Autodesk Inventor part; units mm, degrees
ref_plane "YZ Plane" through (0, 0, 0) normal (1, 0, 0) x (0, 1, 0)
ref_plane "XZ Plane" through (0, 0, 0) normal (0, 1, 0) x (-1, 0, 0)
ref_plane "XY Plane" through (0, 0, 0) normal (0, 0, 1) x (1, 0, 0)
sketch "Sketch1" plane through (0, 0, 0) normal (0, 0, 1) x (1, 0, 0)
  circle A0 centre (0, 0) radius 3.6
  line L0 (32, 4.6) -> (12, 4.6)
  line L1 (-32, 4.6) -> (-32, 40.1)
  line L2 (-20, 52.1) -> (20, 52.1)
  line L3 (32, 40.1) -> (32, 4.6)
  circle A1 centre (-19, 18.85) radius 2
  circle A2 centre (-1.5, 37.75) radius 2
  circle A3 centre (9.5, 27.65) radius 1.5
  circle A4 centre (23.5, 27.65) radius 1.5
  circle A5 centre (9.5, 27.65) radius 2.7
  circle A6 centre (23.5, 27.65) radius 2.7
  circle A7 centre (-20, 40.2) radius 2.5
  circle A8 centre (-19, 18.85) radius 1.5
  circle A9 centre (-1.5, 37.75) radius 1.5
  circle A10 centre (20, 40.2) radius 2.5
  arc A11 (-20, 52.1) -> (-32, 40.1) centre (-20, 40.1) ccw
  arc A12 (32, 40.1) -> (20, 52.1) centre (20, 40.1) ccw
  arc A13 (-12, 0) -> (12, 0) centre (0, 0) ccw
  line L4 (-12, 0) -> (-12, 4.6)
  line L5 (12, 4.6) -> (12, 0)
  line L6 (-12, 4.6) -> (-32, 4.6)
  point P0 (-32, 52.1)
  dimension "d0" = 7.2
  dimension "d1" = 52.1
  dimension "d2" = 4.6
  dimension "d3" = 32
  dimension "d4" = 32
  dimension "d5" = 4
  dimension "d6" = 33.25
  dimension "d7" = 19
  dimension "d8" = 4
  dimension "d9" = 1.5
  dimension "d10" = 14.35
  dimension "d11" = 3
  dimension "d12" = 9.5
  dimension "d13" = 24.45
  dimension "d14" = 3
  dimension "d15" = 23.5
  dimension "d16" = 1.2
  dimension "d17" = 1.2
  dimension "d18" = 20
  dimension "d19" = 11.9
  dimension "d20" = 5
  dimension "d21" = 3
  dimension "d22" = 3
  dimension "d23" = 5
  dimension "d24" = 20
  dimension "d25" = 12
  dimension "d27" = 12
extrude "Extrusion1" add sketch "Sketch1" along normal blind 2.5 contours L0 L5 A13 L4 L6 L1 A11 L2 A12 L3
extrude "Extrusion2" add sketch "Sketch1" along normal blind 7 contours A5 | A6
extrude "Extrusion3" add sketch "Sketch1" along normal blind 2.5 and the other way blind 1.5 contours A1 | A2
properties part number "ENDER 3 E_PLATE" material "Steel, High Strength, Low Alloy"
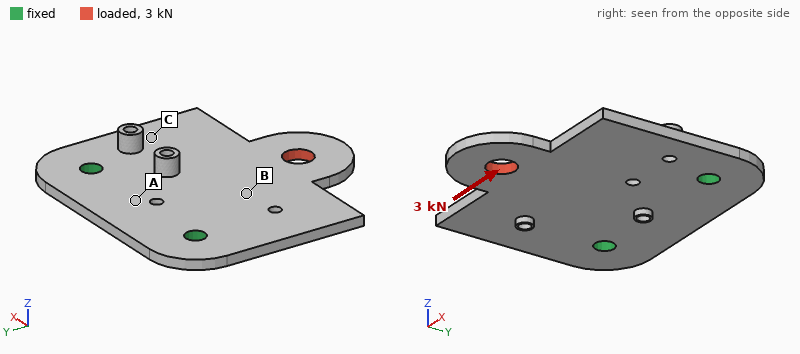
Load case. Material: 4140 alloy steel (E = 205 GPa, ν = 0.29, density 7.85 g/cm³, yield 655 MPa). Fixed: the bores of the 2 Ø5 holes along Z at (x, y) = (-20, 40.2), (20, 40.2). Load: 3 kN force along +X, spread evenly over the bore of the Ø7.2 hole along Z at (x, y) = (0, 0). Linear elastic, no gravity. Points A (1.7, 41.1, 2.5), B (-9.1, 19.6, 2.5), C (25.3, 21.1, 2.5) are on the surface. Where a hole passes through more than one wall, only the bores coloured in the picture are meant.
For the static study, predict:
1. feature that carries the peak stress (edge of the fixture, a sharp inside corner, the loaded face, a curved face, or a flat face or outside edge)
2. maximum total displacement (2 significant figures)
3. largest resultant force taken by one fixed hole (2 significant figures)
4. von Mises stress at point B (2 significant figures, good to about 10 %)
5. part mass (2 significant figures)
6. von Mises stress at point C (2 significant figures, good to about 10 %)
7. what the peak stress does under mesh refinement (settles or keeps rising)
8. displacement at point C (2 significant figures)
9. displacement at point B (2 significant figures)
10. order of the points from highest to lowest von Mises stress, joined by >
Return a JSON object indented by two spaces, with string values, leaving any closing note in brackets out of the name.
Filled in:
{
  "feature that carries the peak stress": "edge of the fixture",
  "maximum total displacement": "34 µm",
  "largest resultant force taken by one fixed hole": "3.2 kN",
  "von Mises stress at point B": "51 MPa",
  "part mass": "64 g",
  "von Mises stress at point C": "34 MPa",
  "what the peak stress does under mesh refinement": "keeps rising",
  "displacement at point C": "11 µm",
  "displacement at point B": "9.9 µm",
  "order of the points from highest to lowest von Mises stress, joined by >": "B > C > A"
}
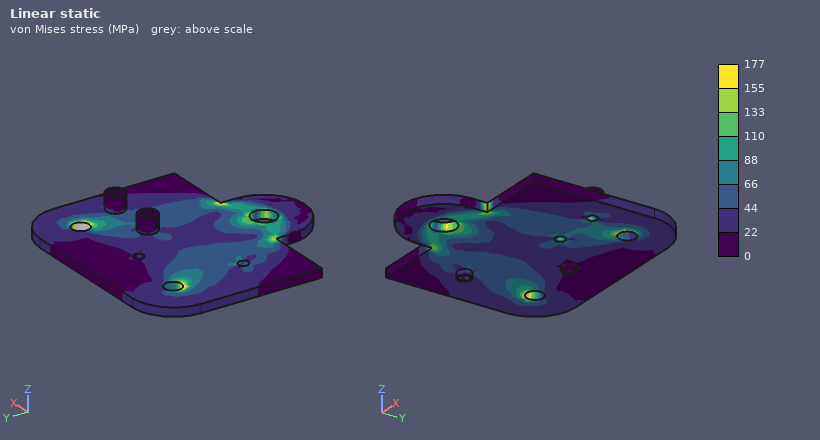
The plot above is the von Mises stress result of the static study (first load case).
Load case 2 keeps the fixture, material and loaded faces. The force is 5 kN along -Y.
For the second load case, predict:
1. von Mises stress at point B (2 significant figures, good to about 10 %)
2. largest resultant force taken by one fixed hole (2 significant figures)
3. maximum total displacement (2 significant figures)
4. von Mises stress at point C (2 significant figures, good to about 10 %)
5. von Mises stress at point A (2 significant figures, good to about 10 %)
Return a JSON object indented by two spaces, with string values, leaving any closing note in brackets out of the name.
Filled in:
{
  "von Mises stress at point B": "56 MPa",
  "largest resultant force taken by one fixed hole": "2.6 kN",
  "maximum total displacement": "18 µm",
  "von Mises stress at point C": "21 MPa",
  "von Mises stress at point A": "14 MPa"
}
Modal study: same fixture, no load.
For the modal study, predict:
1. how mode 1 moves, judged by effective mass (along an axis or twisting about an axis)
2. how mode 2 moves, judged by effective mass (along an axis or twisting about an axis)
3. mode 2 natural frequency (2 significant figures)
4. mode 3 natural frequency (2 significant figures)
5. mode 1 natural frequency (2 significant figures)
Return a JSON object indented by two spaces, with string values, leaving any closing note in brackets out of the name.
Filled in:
{
  "how mode 1 moves, judged by effective mass": "along Z",
  "how mode 2 moves, judged by effective mass": "twisting about Y",
  "mode 2 natural frequency": "2700 Hz",
  "mode 3 natural frequency": "4100 Hz",
  "mode 1 natural frequency": "1100 Hz"
}
